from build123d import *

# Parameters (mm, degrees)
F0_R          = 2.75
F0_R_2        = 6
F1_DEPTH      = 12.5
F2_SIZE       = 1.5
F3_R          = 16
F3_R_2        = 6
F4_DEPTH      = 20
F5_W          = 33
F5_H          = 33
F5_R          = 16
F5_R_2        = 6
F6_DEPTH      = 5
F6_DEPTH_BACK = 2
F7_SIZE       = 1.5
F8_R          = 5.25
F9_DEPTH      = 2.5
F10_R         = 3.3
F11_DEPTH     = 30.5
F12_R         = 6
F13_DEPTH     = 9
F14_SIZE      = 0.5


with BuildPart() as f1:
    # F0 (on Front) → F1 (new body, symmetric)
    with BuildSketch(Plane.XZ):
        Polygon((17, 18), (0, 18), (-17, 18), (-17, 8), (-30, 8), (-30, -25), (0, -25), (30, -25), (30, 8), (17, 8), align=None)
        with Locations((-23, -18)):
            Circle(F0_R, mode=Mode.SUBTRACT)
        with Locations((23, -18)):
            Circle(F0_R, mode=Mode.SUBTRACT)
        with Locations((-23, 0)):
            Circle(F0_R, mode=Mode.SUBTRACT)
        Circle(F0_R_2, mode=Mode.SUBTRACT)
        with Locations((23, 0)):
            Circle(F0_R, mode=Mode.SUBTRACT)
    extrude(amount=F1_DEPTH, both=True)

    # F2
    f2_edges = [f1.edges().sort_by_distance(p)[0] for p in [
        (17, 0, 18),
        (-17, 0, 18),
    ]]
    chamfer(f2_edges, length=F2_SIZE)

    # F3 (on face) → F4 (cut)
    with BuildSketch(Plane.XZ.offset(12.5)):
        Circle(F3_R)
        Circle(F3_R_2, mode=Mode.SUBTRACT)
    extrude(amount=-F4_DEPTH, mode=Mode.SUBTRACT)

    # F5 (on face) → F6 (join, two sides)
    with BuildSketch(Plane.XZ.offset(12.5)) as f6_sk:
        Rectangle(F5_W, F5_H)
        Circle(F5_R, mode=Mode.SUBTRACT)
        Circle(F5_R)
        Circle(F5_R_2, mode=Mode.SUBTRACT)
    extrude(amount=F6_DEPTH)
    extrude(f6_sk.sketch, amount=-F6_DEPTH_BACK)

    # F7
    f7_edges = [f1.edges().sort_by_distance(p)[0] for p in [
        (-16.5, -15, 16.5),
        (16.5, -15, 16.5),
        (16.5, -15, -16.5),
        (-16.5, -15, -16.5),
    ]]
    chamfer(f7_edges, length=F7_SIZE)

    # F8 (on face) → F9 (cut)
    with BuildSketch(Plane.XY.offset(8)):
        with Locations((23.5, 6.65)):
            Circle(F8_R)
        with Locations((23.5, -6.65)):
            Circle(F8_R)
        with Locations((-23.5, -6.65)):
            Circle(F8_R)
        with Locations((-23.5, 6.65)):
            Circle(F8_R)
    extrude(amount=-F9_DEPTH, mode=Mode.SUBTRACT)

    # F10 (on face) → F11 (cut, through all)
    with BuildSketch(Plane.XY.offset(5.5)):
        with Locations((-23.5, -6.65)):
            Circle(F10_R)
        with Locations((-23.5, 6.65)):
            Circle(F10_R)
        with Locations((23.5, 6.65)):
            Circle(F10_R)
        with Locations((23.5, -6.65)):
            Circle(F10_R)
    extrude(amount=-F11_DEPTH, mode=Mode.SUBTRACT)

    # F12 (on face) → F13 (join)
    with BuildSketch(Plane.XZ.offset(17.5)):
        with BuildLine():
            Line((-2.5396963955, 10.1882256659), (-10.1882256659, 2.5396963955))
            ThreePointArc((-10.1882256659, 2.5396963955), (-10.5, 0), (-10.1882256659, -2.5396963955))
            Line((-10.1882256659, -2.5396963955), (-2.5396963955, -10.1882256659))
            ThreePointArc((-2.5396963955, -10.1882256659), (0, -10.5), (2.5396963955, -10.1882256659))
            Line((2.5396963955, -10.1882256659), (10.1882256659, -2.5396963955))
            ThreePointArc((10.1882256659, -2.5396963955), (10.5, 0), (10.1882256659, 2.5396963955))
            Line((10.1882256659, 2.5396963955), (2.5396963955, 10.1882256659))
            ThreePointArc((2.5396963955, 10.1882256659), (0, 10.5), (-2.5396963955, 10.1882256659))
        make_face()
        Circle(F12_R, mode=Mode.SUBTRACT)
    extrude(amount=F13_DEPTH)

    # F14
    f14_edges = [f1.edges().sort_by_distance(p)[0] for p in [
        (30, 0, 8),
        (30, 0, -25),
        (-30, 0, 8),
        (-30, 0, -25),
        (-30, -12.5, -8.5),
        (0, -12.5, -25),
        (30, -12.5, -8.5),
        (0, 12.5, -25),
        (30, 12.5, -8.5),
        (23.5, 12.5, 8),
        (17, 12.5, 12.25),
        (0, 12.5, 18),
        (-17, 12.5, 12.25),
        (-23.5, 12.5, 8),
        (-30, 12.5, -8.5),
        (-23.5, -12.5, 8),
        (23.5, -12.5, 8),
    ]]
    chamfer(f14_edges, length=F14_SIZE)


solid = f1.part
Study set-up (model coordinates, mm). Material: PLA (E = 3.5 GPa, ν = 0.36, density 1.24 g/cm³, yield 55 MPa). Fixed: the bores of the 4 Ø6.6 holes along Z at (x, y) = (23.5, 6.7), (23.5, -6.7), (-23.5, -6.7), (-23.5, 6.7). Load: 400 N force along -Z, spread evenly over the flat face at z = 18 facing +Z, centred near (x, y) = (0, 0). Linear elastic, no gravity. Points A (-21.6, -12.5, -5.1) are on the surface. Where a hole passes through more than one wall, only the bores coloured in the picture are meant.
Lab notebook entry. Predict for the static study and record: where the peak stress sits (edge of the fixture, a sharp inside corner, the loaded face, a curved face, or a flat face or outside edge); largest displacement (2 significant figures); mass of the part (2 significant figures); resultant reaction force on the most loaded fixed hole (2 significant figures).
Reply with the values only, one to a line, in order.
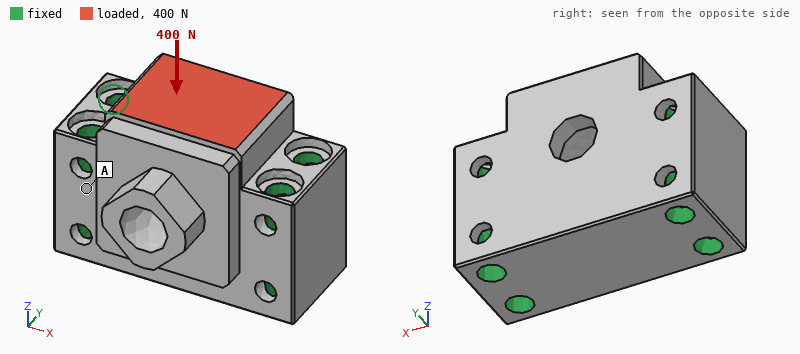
the loaded face
31 µm
53 g
120 N
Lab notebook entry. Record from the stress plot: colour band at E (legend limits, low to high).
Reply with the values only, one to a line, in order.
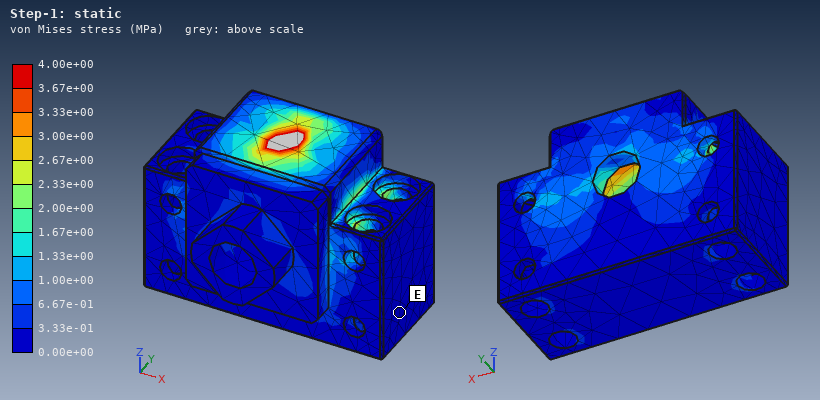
0.00e+00 to 3.33e-01 MPa
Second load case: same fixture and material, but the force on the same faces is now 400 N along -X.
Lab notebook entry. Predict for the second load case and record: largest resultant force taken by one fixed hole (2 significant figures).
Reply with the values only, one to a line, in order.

130 N
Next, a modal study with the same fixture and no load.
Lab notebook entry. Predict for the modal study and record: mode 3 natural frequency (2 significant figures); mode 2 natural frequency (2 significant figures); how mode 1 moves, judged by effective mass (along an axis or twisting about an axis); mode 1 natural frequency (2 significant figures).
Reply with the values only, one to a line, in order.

8800 Hz
8700 Hz
along Y
5600 Hz
